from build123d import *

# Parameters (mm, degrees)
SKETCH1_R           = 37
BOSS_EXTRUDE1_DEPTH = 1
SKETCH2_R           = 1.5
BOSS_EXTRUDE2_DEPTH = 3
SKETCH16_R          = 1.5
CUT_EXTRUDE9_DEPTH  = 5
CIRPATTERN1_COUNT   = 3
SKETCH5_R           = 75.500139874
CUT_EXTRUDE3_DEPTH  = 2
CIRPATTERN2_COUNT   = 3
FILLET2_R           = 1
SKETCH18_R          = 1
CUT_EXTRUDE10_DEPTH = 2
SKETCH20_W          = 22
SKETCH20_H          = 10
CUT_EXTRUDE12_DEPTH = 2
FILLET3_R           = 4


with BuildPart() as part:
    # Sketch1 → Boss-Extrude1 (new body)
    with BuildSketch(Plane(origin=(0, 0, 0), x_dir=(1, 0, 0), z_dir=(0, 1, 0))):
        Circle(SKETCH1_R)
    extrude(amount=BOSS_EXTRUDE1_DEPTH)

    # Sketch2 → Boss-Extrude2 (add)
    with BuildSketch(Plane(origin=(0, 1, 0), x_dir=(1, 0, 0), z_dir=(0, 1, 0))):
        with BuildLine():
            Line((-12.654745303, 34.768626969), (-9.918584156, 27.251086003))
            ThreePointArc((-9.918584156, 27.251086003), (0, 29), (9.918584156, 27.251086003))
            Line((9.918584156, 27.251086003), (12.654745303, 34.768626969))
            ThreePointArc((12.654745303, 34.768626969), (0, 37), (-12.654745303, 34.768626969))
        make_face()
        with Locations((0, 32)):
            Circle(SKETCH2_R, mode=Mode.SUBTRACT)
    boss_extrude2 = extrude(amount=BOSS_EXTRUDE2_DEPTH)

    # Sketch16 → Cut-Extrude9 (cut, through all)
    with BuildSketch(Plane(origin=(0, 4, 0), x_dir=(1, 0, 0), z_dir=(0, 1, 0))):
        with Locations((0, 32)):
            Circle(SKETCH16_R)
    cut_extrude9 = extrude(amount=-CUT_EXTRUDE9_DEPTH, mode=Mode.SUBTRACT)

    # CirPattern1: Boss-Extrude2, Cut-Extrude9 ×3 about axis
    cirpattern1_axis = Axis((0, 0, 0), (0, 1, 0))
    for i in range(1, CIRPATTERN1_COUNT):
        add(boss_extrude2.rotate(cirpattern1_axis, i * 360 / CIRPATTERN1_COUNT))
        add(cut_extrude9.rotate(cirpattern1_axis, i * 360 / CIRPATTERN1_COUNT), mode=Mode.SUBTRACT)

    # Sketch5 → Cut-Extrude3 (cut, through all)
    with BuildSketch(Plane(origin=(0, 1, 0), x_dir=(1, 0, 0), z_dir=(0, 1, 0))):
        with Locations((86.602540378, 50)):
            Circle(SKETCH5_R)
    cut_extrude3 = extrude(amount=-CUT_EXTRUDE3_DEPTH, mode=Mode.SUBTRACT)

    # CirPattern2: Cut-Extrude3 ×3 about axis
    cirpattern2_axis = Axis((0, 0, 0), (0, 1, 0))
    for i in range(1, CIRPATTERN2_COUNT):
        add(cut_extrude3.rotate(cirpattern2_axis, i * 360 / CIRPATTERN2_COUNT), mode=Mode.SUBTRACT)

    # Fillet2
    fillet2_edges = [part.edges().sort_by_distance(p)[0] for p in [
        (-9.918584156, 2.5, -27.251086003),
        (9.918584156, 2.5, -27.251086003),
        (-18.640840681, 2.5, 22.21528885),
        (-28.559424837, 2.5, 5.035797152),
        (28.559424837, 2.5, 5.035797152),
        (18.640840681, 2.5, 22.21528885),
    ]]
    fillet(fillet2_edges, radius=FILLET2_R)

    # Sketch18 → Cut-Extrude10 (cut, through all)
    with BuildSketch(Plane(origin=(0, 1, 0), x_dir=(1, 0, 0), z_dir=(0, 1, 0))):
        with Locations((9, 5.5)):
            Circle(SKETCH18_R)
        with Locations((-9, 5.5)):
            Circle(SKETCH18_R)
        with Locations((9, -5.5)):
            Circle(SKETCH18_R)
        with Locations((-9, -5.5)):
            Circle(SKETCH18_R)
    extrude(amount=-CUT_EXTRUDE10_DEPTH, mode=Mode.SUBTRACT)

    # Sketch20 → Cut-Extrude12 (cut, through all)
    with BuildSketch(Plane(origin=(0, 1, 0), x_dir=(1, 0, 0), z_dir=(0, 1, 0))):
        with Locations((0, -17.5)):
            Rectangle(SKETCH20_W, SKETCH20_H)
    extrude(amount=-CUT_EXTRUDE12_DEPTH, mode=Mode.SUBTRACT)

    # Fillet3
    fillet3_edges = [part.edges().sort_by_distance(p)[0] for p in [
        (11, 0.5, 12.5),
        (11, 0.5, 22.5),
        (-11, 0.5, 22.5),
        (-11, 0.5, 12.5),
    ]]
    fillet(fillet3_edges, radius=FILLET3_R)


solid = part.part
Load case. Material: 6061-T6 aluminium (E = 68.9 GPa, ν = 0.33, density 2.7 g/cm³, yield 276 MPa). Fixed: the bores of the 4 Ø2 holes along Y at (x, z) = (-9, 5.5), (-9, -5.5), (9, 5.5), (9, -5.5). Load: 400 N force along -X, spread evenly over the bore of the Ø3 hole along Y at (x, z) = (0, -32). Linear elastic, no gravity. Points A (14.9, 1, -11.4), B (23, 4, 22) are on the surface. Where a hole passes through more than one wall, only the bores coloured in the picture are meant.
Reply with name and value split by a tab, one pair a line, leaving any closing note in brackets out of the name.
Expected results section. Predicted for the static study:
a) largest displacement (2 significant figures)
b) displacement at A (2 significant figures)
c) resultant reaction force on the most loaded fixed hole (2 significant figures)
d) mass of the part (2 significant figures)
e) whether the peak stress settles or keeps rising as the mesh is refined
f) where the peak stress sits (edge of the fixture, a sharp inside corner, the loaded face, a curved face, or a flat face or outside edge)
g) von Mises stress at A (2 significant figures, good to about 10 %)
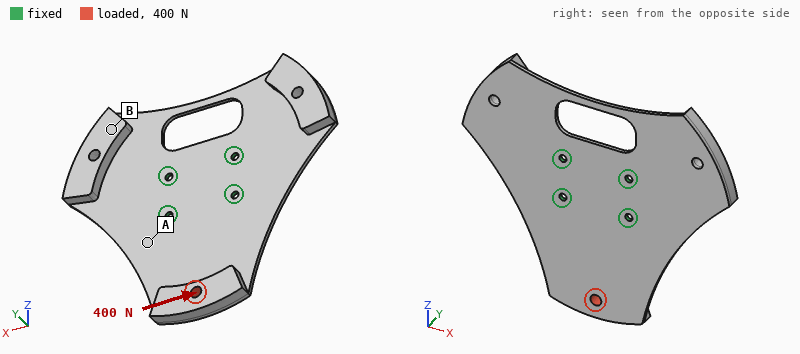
largest displacement	0.28 mm
displacement at A	0.057 mm
resultant reaction force on the most loaded fixed hole	420 N
mass of the part	12 g
whether the peak stress settles or keeps rising as the mesh is refined	keeps rising
where the peak stress sits	edge of the fixture
von Mises stress at A	24 MPa
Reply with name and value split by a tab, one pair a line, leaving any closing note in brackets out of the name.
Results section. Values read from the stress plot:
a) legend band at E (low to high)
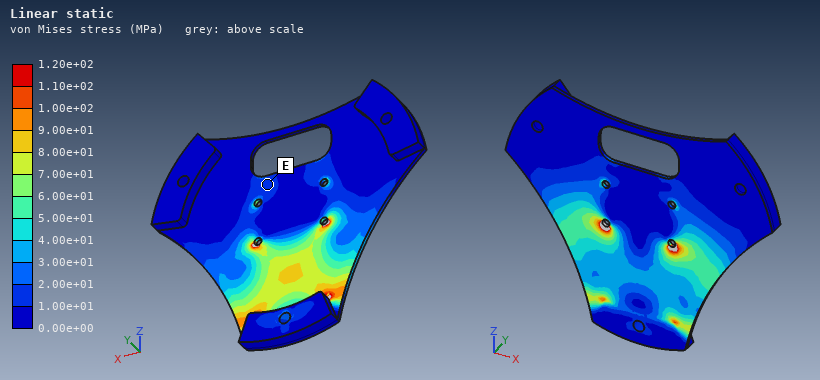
legend band at E	1.00e+01 to 2.00e+01 MPa
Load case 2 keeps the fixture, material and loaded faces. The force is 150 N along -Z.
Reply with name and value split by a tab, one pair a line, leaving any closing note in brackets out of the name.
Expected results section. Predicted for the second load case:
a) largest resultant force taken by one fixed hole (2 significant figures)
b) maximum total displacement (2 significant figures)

largest resultant force taken by one fixed hole	56 N
maximum total displacement	0.48 mm
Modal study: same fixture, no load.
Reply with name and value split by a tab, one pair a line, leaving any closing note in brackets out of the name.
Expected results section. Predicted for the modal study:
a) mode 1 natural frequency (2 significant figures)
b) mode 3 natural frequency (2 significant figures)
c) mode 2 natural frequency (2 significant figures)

mode 1 natural frequency	610 Hz
mode 3 natural frequency	690 Hz
mode 2 natural frequency	680 Hz
